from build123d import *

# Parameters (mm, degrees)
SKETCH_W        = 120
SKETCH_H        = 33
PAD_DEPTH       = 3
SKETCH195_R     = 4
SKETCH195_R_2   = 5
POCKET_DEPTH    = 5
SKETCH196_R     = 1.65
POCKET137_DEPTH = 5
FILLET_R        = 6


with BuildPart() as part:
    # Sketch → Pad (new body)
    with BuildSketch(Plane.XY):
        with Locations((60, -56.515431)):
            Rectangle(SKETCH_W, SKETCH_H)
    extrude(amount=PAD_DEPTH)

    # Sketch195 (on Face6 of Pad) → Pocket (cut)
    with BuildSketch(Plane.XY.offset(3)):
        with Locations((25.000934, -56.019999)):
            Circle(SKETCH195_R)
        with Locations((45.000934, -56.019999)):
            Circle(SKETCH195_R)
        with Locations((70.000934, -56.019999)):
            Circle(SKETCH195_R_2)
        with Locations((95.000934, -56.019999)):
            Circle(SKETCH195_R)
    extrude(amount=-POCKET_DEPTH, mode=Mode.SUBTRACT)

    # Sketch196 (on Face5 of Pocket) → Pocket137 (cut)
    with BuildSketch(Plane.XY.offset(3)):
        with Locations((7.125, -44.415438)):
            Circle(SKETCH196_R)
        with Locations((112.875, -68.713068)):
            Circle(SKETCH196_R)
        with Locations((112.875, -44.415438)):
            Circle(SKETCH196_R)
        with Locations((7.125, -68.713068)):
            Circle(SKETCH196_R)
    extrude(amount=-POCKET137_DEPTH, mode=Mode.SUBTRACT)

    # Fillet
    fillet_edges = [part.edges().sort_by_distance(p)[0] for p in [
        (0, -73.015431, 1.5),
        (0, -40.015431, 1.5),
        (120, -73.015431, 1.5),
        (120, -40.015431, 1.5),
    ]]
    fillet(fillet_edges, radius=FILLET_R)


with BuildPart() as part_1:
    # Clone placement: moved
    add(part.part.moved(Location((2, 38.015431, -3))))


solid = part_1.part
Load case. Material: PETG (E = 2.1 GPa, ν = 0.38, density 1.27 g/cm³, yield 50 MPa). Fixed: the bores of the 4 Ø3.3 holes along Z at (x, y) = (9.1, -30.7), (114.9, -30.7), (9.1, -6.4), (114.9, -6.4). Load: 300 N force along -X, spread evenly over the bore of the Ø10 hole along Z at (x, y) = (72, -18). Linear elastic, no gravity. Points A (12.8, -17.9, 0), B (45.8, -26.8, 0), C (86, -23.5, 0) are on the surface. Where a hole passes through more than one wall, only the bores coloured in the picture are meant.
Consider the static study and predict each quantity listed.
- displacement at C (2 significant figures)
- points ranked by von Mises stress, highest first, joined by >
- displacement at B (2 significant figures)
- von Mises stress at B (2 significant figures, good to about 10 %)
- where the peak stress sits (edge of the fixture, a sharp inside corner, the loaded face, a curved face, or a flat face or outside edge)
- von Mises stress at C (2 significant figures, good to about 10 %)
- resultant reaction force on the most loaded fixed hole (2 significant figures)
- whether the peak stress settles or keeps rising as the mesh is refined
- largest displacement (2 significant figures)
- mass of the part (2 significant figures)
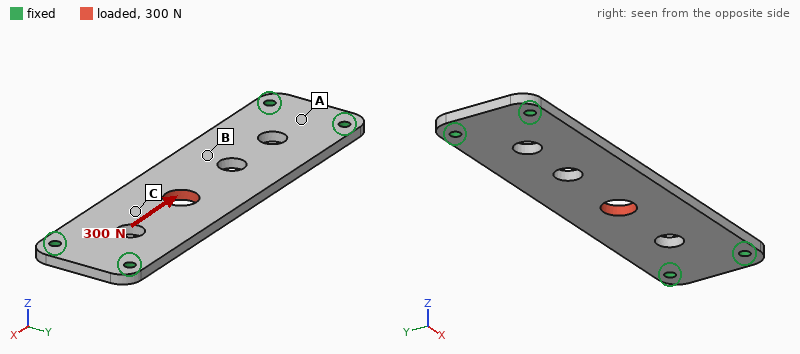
35 µm
C > B > A
28 µm
1.5 MPa
edge of the fixture
2.5 MPa
90 N
keeps rising
53 µm
14 g
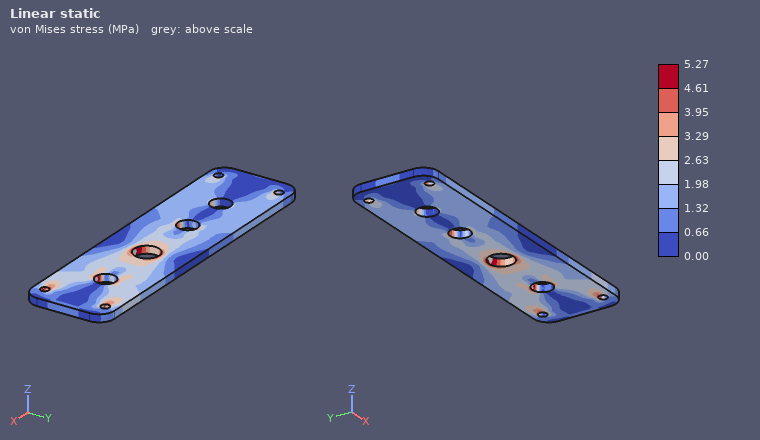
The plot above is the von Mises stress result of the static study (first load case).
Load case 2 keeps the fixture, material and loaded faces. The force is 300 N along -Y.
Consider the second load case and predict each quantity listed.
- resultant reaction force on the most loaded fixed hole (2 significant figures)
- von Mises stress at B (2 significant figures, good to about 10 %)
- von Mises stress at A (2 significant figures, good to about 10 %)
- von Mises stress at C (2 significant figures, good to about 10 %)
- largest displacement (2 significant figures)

190 N
3.6 MPa
2.1 MPa
4.4 MPa
0.25 mm
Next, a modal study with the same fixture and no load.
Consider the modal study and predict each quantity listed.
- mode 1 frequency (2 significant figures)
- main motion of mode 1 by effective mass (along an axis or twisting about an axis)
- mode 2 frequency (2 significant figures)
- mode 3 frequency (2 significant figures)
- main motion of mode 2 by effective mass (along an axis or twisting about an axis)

350 Hz
along Z
760 Hz
960 Hz
twisting about X
